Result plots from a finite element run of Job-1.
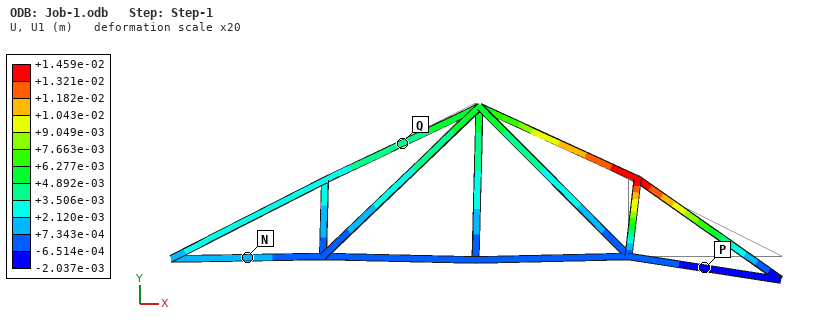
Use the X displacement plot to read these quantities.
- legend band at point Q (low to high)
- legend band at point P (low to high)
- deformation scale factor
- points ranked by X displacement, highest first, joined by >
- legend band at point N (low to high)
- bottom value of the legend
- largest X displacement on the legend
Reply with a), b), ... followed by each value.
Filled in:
a) +3.506e-03 to +4.892e-03 m
b) -2.037e-03 to -6.514e-04 m
c) 20
d) Q > N > P
e) +7.343e-04 to +2.120e-03 m
f) -2.037e-03 m
g) +1.459e-02 m
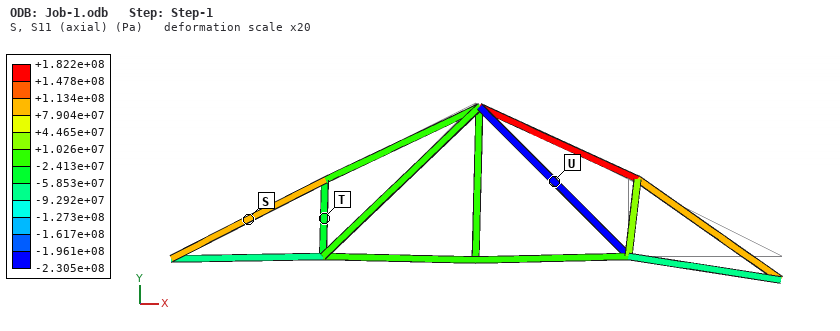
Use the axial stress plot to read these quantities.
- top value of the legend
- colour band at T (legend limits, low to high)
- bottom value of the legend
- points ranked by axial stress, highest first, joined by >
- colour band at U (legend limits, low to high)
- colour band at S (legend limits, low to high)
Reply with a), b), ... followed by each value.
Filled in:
a) +1.822e+08 Pa
b) -5.853e+07 to -2.413e+07 Pa
c) -2.305e+08 Pa
d) S > T > U
e) -2.305e+08 to -1.961e+08 Pa
f) +7.904e+07 to +1.134e+08 Pa
